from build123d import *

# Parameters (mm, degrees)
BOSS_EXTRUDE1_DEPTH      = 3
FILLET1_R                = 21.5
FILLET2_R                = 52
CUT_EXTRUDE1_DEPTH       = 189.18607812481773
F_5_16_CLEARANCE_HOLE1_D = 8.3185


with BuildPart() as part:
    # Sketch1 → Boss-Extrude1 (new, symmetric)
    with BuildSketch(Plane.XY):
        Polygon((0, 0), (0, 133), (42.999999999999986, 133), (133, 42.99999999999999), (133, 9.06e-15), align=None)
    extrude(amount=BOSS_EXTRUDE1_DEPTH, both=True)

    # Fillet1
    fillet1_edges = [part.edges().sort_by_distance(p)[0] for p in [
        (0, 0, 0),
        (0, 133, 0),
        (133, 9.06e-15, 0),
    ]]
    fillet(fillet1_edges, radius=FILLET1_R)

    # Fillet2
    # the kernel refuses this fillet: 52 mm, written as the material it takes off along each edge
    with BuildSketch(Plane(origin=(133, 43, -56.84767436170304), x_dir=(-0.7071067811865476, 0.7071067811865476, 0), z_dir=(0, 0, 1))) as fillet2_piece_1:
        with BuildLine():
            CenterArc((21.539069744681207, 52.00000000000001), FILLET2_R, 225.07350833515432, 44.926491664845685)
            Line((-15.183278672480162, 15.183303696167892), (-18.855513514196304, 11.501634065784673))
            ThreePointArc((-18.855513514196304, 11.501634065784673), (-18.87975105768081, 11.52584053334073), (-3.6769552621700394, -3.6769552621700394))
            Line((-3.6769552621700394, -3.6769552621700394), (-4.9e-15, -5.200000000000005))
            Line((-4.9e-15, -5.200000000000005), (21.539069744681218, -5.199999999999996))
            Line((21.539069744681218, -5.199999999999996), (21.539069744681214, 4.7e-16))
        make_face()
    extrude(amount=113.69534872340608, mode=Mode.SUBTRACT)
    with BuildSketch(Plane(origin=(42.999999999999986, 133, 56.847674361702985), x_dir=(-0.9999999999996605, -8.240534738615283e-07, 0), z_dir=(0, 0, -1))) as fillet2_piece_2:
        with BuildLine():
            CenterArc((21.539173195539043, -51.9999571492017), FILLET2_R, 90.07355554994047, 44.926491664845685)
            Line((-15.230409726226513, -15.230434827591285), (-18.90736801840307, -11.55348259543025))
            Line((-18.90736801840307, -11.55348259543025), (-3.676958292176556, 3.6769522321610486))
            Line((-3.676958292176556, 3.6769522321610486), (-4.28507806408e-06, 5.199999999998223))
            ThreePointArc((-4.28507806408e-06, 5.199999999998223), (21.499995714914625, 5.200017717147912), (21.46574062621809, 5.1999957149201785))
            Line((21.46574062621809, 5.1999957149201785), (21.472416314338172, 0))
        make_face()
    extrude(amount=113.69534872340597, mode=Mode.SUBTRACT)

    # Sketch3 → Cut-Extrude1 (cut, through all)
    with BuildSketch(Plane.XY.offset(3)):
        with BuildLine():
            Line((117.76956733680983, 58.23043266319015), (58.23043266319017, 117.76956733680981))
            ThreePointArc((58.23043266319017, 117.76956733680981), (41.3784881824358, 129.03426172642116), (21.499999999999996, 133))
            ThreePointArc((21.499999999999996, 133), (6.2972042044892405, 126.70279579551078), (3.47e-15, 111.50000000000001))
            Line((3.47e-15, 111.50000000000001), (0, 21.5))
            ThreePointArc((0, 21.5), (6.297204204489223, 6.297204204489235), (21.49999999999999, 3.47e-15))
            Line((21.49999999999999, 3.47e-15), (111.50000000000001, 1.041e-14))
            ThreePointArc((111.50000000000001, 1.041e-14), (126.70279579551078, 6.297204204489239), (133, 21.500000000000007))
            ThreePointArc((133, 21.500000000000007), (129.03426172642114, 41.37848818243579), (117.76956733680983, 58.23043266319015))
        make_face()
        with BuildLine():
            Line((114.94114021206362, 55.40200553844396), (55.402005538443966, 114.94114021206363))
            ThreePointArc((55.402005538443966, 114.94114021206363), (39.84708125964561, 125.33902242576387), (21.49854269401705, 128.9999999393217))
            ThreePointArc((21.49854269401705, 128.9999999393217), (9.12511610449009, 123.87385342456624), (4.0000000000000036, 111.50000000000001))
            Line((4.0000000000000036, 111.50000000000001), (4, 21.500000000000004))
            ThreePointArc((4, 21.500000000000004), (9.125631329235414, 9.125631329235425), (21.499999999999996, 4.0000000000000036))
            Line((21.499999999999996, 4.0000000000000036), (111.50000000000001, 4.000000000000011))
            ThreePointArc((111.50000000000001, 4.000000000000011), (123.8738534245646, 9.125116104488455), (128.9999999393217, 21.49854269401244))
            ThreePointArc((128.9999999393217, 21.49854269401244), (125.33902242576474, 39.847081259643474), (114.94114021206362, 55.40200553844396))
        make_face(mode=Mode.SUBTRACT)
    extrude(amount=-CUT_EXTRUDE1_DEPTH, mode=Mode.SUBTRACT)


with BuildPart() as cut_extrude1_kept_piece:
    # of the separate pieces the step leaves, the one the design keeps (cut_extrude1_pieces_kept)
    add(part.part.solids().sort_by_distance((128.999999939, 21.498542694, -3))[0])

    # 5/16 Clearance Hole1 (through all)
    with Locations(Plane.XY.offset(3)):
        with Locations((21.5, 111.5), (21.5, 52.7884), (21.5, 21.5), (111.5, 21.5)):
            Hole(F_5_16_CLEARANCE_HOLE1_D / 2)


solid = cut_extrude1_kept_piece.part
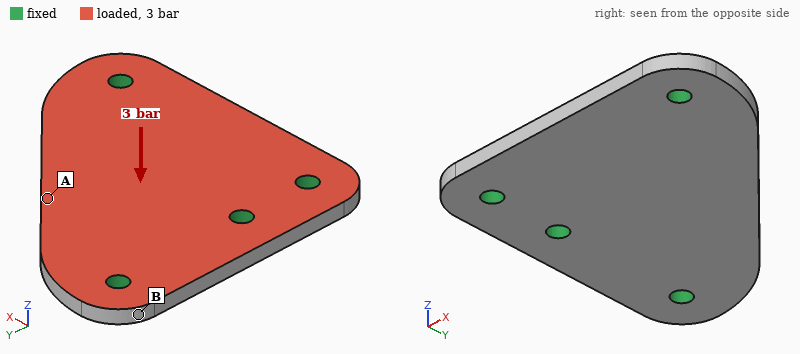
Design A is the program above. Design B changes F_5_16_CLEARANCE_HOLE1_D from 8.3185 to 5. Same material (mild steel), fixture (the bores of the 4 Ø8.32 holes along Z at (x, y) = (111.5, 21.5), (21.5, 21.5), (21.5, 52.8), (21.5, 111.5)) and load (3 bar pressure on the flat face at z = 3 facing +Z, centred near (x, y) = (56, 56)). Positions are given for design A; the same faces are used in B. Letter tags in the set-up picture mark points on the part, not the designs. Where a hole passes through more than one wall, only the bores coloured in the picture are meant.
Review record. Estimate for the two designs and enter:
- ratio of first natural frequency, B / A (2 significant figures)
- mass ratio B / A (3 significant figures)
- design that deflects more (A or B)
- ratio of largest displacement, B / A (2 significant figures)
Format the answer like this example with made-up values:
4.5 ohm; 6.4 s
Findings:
0.91; 1.01; B; 1.2
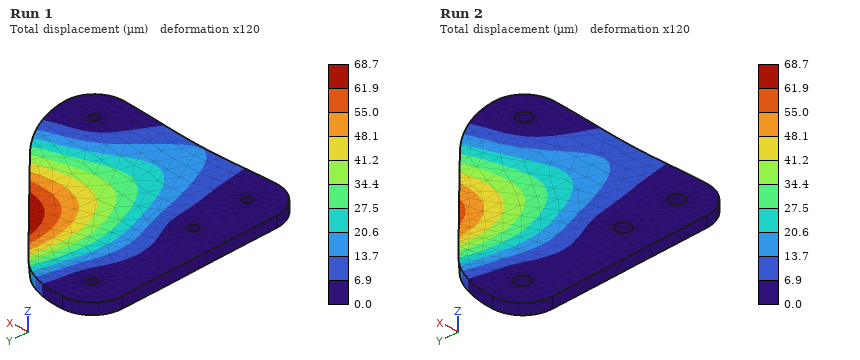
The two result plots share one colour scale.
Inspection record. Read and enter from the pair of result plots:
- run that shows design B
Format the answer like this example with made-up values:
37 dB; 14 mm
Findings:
Run 1
